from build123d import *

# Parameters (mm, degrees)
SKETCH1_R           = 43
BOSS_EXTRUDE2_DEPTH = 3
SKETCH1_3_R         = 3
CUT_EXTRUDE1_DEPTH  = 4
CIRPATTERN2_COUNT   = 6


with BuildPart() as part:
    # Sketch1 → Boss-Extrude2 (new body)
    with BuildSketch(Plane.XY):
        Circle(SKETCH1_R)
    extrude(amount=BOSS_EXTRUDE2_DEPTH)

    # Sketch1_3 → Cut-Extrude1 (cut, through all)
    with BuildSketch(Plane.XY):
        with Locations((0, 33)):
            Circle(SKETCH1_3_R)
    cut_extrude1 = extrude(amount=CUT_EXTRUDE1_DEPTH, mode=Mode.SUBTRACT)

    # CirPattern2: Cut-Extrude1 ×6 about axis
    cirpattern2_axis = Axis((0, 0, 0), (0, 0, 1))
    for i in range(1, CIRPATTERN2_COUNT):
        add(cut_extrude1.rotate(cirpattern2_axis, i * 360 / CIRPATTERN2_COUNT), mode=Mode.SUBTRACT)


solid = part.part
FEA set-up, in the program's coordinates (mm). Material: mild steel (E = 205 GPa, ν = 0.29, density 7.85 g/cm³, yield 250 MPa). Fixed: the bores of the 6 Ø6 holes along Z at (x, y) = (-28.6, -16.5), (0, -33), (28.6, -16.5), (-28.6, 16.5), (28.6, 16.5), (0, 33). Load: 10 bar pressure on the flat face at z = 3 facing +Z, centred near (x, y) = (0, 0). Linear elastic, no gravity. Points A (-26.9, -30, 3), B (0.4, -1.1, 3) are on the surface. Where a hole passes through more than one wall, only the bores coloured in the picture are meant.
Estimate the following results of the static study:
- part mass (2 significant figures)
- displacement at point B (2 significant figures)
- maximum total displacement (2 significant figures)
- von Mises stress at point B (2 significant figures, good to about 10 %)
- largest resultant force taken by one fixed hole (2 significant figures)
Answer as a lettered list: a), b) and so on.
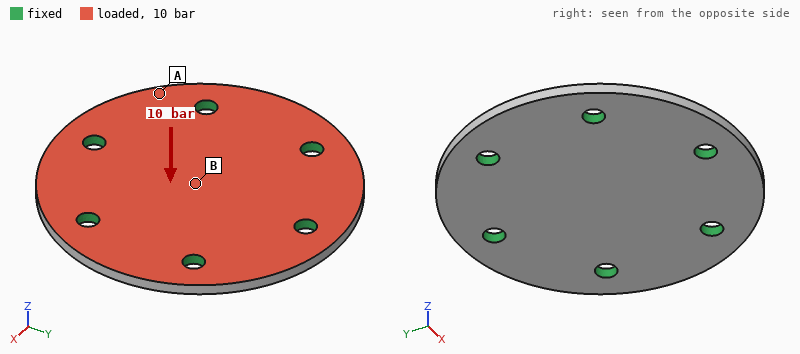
a) 130 g
b) 36 µm
c) 36 µm
d) 54 MPa
e) 940 N
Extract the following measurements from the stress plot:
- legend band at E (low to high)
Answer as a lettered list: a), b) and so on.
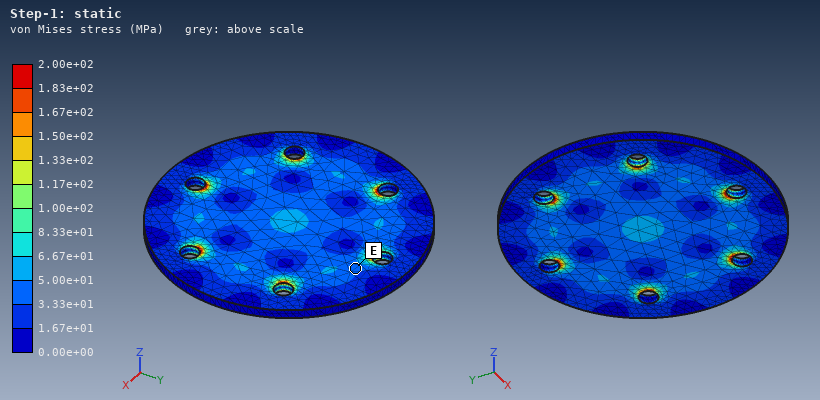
a) 3.33e+01 to 5.00e+01 MPa
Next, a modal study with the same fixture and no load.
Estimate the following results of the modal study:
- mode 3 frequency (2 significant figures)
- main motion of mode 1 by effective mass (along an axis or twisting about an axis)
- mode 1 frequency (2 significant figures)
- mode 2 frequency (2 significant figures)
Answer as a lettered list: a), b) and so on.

a) 12 kHz
b) along Z
c) 6600 Hz
d) 11 kHz
